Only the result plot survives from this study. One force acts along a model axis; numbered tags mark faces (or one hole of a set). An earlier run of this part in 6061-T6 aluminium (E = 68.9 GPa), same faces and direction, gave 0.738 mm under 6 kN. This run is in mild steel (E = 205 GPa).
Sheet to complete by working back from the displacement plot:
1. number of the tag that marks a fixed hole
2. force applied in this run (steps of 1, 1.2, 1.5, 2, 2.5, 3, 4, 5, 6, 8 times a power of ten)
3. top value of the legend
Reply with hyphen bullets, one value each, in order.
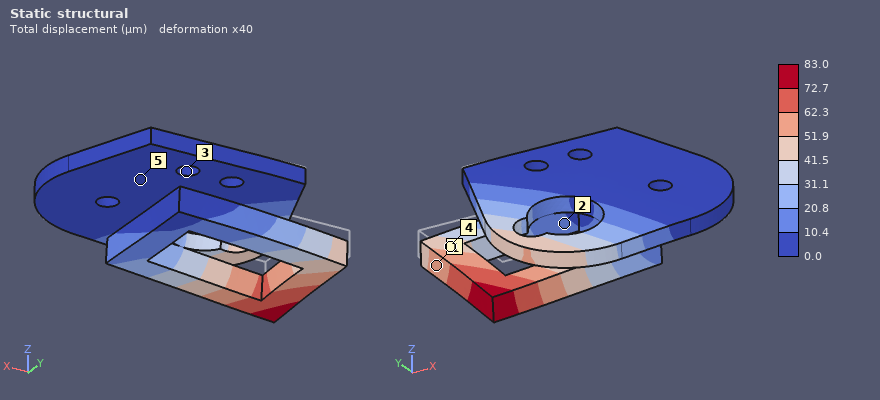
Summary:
- 3
- 2 kN
- 83.0 µm
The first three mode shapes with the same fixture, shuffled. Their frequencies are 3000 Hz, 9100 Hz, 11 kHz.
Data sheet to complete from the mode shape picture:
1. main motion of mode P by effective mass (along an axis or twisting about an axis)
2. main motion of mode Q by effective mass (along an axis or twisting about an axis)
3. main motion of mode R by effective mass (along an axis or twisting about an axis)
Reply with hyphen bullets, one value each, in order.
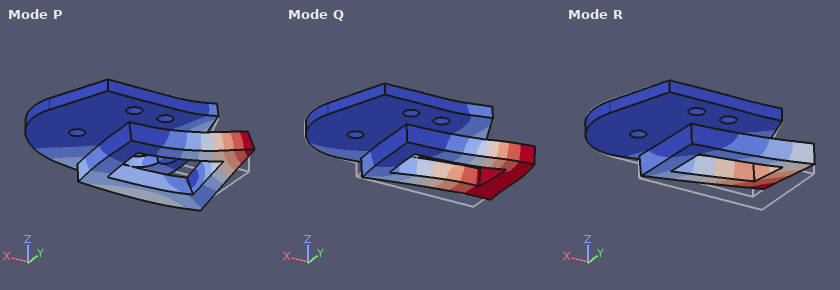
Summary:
- twisting about X
- along Y
- along Z
